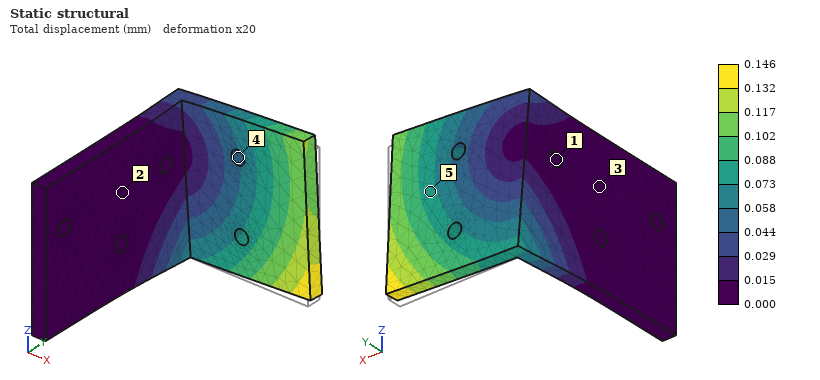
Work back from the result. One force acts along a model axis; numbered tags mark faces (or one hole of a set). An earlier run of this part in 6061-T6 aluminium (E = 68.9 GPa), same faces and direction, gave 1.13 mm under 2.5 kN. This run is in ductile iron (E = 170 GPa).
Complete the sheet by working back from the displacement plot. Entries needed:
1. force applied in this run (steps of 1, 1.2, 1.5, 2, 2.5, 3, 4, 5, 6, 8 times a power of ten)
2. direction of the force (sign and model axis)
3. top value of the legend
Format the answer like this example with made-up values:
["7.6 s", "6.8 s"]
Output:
["800 N", "+Z", "0.146 mm"]
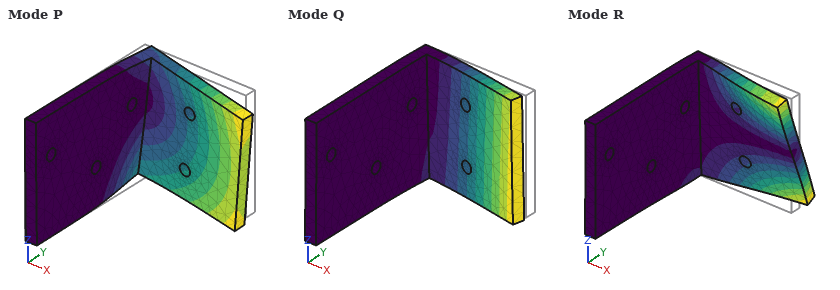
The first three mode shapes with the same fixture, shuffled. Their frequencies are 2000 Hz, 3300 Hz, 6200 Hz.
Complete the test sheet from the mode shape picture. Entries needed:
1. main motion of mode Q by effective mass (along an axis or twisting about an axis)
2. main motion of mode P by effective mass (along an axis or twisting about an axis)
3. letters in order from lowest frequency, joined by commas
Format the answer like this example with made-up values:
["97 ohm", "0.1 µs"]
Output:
["along Y", "along Z", "Q, P, R"]
